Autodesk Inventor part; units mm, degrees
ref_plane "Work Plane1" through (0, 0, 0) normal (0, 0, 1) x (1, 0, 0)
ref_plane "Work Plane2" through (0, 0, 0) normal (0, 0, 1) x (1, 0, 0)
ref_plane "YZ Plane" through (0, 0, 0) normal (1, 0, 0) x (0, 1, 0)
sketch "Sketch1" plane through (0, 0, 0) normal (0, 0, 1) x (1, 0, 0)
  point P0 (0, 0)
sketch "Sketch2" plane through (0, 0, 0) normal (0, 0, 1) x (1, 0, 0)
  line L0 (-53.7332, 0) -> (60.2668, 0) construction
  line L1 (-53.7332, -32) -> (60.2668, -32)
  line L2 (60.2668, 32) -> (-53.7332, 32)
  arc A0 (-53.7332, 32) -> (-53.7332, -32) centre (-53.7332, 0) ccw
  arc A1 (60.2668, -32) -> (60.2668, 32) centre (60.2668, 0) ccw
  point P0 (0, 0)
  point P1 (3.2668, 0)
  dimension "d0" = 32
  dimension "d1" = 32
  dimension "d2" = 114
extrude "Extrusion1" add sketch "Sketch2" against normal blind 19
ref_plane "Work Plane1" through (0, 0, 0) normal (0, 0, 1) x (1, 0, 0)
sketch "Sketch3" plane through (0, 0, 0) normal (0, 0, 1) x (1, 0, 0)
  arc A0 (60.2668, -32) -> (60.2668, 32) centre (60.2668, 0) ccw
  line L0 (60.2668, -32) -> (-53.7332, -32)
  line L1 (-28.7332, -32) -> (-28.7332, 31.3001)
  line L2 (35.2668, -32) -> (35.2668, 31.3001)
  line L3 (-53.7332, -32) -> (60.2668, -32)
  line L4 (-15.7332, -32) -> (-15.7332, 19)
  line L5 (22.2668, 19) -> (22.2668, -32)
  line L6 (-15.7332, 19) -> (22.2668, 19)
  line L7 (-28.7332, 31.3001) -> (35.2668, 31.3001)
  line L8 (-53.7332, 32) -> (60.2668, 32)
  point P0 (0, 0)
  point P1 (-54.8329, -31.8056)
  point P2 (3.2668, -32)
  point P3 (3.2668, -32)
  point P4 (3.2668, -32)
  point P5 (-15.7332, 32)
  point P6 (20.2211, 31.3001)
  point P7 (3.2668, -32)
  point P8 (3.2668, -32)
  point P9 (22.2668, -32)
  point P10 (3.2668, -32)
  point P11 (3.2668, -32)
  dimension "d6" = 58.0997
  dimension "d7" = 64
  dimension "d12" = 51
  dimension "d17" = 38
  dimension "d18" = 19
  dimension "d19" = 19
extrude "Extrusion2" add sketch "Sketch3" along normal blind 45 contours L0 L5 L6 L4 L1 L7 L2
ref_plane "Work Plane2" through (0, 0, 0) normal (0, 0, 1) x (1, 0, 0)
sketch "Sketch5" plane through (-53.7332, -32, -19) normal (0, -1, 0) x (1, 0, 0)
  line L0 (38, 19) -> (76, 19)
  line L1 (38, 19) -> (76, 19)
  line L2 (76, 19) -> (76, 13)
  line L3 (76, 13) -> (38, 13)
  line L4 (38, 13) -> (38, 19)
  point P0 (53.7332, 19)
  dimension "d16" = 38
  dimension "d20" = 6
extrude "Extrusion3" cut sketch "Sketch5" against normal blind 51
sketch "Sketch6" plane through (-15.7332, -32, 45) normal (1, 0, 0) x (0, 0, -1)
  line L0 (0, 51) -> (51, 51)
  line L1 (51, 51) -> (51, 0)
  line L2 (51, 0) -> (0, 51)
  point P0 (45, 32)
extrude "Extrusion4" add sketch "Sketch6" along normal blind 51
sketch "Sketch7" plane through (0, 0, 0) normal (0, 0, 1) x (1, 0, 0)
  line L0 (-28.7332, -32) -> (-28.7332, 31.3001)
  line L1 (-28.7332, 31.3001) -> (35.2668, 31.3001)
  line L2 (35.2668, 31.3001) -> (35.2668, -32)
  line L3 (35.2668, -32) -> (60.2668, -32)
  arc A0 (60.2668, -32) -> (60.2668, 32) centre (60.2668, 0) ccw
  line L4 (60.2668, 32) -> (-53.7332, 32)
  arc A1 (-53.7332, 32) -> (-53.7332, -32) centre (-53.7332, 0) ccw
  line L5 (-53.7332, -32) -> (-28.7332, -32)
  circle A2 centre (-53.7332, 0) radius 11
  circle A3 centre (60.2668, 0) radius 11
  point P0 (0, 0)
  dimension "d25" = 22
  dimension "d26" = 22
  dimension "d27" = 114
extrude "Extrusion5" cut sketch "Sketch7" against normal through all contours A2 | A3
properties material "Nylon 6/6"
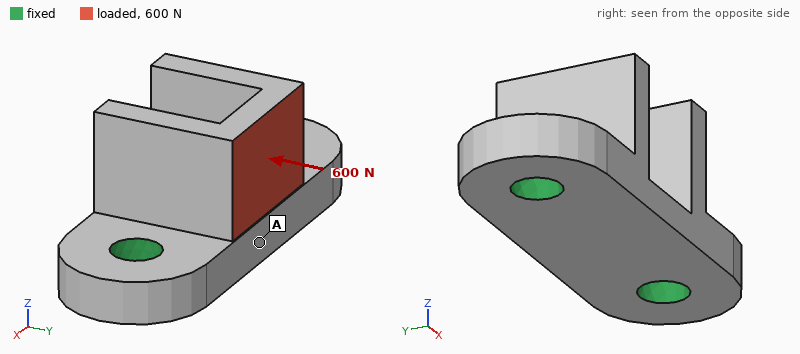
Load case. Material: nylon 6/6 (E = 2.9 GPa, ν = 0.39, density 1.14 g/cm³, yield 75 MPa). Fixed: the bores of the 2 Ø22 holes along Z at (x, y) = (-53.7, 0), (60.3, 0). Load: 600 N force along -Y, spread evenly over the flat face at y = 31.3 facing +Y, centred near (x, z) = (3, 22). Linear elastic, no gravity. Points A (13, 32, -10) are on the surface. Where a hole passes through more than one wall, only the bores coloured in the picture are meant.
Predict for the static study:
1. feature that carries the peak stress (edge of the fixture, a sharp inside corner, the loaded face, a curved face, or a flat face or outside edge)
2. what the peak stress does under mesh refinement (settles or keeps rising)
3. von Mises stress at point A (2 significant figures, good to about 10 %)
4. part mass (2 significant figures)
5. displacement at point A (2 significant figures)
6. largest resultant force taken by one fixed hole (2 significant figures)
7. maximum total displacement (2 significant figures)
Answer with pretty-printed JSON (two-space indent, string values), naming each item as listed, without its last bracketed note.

{
  "feature that carries the peak stress": "edge of the fixture",
  "what the peak stress does under mesh refinement": "keeps rising",
  "von Mises stress at point A": "0.48 MPa",
  "part mass": "360 g",
  "displacement at point A": "0.047 mm",
  "largest resultant force taken by one fixed hole": "300 N",
  "maximum total displacement": "0.11 mm"
}
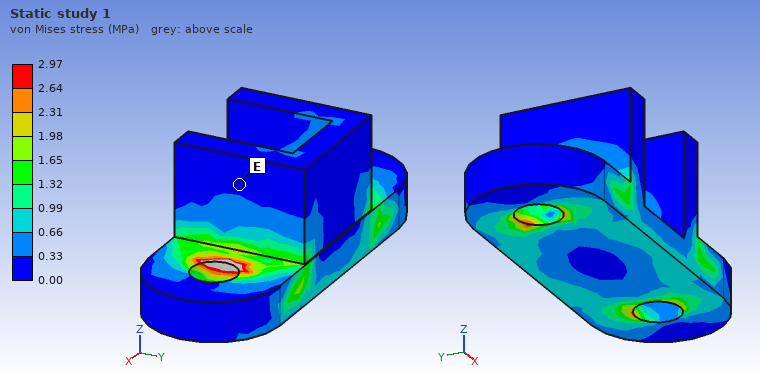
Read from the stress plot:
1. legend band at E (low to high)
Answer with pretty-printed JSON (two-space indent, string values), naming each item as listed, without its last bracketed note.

{
  "legend band at E": "0.00 to 0.33 MPa"
}
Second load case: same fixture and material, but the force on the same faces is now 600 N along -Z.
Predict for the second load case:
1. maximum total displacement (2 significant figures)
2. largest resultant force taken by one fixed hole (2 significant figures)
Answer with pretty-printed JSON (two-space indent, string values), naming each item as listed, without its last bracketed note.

{
  "maximum total displacement": "0.10 mm",
  "largest resultant force taken by one fixed hole": "330 N"
}
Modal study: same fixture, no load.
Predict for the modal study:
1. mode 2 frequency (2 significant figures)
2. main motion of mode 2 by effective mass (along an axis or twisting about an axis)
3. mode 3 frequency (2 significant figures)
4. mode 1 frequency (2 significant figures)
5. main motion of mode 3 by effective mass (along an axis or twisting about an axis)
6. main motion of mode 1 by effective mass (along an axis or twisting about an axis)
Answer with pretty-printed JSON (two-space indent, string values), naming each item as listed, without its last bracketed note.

{
  "mode 2 frequency": "2000 Hz",
  "main motion of mode 2 by effective mass": "along Z",
  "mode 3 frequency": "2200 Hz",
  "mode 1 frequency": "1100 Hz",
  "main motion of mode 3 by effective mass": "along X",
  "main motion of mode 1 by effective mass": "along Y"
}
